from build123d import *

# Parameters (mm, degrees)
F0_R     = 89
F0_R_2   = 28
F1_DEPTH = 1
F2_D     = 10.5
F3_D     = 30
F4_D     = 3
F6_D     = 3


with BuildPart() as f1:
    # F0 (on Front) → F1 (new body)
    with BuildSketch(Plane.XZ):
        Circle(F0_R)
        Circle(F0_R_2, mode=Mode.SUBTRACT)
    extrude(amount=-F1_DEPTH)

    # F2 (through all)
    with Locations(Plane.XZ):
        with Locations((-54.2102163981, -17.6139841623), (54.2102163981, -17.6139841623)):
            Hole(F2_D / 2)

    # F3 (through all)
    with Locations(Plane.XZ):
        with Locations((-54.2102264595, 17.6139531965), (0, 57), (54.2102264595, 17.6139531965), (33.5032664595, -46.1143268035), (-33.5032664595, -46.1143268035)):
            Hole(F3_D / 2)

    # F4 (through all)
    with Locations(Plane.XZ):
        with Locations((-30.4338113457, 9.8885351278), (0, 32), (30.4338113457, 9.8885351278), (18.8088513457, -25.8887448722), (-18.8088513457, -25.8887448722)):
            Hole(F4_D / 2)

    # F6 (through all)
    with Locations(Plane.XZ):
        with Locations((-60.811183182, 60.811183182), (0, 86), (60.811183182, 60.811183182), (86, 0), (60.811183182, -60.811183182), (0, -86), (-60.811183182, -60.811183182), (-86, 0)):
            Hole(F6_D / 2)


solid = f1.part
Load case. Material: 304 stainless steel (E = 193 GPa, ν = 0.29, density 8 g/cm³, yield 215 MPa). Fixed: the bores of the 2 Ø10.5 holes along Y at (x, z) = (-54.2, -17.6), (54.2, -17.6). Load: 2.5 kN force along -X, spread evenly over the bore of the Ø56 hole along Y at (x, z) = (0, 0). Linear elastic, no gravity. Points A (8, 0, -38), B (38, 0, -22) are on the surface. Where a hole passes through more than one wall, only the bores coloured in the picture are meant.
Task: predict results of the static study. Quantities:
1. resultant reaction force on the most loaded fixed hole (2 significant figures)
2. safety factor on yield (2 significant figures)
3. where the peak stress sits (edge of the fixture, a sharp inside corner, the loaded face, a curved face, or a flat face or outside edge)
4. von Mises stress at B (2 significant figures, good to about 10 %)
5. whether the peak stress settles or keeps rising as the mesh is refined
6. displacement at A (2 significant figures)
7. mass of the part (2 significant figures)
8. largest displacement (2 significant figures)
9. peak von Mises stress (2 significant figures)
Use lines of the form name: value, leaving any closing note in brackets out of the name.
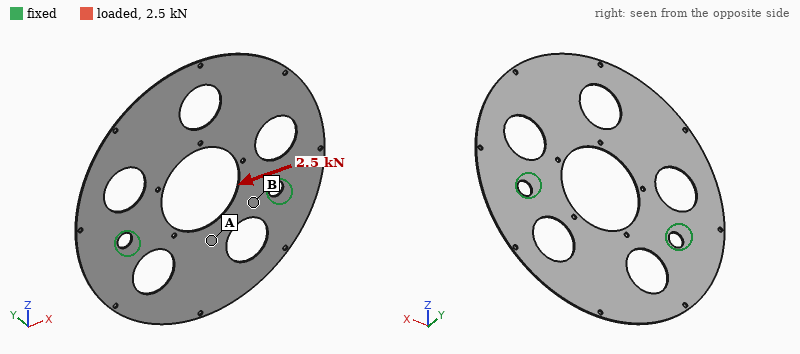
resultant reaction force on the most loaded fixed hole: 1.3 kN
safety factor on yield: 1.4
where the peak stress sits: a curved face
von Mises stress at B: 27 MPa
whether the peak stress settles or keeps rising as the mesh is refined: settles
displacement at A: 4.7 µm
mass of the part: 150 g
largest displacement: 27 µm
peak von Mises stress: 160 MPa
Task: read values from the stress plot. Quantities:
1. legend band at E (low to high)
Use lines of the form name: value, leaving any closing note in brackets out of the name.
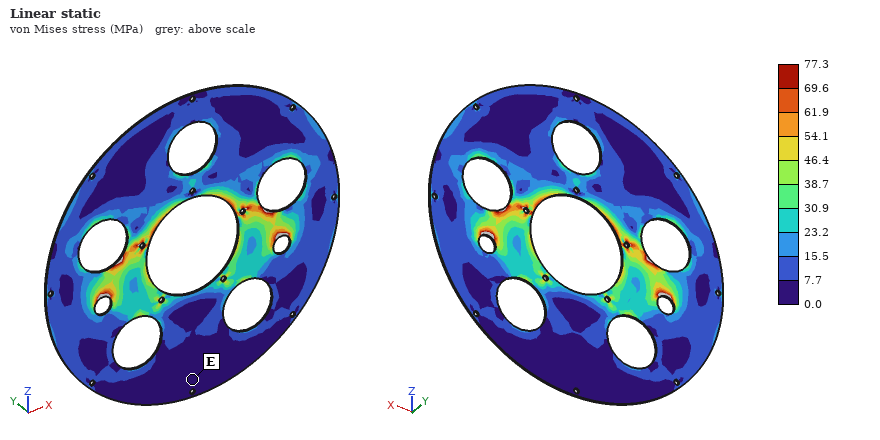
legend band at E: 0.0 to 7.7 MPa
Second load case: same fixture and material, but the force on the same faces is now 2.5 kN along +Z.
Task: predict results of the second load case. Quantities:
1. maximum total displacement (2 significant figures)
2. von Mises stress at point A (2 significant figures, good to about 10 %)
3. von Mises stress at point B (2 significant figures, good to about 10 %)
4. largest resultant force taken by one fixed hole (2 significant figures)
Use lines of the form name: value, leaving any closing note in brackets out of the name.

maximum total displacement: 15 µm
von Mises stress at point A: 20 MPa
von Mises stress at point B: 37 MPa
largest resultant force taken by one fixed hole: 1.3 kN
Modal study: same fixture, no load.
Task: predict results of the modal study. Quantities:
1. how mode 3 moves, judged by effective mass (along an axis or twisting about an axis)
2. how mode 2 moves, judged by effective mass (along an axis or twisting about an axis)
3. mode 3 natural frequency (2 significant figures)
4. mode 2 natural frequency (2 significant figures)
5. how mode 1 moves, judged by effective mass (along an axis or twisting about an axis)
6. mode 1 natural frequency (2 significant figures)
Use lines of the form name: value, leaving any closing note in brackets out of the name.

how mode 3 moves, judged by effective mass: twisting about Z
how mode 2 moves, judged by effective mass: along Y
mode 3 natural frequency: 180 Hz
mode 2 natural frequency: 160 Hz
how mode 1 moves, judged by effective mass: along Y
mode 1 natural frequency: 70 Hz
